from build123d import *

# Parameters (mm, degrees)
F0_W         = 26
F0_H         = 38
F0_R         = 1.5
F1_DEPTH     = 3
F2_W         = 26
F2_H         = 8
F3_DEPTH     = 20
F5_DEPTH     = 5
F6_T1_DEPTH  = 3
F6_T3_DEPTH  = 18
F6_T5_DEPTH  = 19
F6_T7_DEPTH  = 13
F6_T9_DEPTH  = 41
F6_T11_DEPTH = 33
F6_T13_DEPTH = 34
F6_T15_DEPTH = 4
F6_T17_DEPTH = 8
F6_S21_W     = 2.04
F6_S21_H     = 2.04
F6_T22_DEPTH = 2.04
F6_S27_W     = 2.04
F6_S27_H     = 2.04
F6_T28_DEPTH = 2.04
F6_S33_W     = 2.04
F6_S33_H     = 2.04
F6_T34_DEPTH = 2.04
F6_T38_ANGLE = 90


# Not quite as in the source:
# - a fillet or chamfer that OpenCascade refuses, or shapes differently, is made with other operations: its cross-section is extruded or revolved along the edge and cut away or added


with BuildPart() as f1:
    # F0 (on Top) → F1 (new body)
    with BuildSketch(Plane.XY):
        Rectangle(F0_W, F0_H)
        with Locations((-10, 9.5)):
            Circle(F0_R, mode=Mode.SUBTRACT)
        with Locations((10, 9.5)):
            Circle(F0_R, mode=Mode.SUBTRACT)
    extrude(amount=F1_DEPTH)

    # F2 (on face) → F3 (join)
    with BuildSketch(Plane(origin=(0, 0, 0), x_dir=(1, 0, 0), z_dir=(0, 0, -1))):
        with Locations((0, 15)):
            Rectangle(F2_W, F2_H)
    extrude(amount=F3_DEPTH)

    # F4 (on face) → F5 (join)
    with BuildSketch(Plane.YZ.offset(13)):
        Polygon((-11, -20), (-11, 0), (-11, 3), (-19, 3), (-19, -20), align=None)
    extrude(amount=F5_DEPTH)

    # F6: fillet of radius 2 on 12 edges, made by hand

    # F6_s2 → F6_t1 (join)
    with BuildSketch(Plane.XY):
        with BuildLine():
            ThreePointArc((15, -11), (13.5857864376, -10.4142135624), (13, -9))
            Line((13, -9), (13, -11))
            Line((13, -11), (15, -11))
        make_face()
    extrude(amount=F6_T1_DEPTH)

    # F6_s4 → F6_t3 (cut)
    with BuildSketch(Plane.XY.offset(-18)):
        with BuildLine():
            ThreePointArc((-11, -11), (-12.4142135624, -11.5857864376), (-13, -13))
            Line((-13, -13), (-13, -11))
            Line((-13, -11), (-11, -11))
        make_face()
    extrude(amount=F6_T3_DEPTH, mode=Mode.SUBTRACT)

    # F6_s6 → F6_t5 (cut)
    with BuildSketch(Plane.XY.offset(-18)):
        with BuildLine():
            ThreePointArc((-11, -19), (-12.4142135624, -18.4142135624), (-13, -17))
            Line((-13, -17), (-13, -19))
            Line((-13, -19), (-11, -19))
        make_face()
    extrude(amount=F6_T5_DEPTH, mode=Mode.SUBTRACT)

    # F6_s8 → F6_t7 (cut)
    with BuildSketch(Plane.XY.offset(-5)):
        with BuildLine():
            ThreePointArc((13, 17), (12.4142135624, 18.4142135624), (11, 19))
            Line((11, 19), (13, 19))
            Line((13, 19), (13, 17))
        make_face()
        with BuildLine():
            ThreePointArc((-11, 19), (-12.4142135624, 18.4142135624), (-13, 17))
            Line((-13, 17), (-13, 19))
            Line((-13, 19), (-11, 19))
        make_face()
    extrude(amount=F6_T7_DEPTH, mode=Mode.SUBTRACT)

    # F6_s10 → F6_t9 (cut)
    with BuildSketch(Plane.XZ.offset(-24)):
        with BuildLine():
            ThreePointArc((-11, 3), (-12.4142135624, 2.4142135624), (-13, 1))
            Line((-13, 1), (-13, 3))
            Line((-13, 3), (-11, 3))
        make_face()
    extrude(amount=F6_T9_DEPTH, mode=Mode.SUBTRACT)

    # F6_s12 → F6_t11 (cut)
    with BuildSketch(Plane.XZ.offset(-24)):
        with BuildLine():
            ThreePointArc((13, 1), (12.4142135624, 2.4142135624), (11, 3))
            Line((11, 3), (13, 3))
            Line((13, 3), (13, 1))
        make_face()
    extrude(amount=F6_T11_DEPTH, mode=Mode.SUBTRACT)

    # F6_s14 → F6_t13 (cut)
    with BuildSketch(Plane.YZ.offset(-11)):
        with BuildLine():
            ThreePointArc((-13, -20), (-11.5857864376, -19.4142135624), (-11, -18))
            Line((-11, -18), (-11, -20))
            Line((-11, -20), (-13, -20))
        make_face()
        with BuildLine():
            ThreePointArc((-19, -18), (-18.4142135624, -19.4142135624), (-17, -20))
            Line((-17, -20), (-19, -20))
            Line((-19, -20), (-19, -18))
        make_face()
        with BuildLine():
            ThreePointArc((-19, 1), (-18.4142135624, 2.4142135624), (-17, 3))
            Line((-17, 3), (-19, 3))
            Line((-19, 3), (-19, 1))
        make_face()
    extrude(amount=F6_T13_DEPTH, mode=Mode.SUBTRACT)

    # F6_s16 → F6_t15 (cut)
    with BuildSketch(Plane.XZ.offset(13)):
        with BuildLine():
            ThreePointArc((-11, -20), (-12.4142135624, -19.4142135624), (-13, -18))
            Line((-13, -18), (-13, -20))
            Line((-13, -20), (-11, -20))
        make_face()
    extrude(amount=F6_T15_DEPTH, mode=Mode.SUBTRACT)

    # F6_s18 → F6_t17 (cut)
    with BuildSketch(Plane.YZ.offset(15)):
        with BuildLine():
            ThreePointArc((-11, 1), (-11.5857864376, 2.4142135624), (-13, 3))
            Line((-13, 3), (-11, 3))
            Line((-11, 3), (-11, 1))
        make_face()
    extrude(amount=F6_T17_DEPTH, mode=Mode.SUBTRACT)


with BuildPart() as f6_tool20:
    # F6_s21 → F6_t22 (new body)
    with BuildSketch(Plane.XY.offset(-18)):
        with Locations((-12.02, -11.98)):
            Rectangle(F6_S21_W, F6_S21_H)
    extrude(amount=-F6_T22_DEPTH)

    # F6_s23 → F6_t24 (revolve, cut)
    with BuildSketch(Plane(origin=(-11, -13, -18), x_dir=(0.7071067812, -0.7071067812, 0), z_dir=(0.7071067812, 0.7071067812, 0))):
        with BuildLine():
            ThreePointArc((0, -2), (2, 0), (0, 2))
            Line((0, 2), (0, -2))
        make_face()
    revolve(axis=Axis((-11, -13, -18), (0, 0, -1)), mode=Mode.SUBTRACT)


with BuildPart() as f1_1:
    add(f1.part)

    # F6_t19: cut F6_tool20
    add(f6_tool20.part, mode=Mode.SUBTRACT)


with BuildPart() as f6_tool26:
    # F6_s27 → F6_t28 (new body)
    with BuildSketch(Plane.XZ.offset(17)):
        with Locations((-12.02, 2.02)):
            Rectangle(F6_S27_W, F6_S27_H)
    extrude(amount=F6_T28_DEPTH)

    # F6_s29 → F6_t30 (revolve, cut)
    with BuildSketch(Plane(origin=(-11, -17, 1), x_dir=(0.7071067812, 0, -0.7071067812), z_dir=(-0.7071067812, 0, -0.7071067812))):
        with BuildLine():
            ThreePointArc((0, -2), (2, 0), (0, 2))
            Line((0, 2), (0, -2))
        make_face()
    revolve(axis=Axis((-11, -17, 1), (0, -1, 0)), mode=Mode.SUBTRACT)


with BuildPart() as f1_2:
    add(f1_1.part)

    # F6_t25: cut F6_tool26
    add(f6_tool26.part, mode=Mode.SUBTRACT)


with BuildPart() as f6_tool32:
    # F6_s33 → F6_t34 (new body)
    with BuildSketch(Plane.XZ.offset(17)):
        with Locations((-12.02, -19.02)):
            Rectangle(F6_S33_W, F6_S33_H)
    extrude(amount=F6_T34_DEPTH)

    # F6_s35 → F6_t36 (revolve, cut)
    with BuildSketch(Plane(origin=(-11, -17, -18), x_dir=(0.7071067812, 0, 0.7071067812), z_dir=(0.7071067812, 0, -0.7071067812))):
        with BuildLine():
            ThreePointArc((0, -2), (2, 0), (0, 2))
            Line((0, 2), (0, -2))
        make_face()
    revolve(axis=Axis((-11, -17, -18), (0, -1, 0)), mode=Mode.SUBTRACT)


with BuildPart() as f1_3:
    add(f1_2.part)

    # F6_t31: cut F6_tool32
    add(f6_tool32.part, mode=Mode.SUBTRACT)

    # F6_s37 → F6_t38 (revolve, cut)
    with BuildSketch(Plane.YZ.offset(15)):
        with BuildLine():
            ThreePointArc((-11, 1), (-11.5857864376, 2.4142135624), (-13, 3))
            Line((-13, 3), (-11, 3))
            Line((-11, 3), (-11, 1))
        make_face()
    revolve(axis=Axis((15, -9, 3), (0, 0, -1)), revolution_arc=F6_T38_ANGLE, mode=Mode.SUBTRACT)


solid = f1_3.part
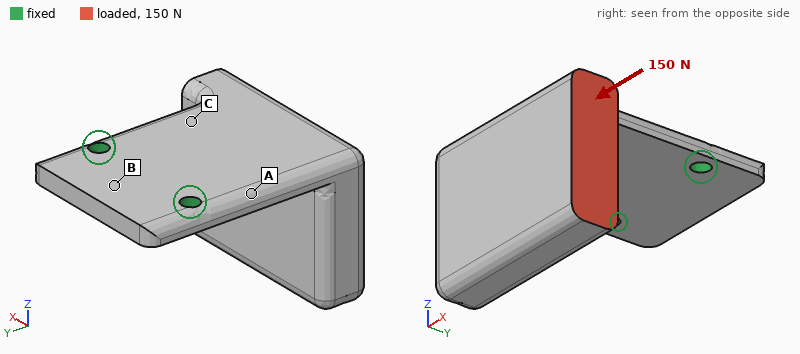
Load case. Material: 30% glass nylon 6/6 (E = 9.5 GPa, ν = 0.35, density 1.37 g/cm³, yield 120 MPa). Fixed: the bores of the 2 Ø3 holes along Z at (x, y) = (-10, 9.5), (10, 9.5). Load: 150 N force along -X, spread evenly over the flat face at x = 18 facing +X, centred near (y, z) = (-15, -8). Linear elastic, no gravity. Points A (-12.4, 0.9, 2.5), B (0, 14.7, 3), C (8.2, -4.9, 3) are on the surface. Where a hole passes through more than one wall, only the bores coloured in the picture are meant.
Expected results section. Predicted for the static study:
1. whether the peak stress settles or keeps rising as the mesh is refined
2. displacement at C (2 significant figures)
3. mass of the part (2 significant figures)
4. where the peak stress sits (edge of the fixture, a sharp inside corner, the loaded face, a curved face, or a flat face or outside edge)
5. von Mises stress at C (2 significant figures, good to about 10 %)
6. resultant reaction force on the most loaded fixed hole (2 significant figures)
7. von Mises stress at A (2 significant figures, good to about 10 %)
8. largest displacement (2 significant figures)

keeps rising
0.12 mm
11 g
edge of the fixture
20 MPa
210 N
22 MPa
0.61 mm
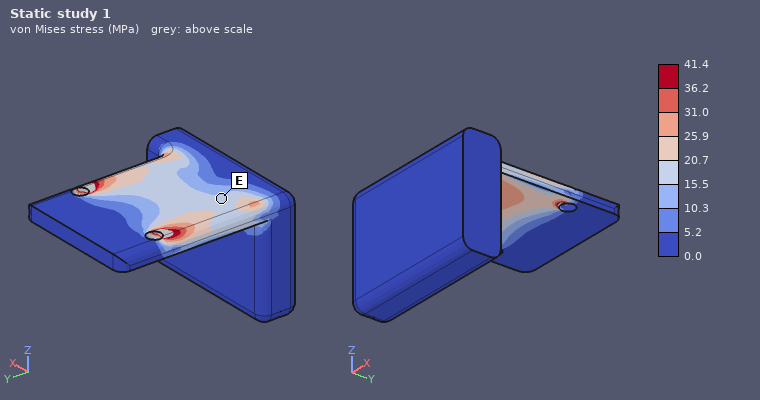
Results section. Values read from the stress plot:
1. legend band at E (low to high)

15.5 to 20.7 MPa
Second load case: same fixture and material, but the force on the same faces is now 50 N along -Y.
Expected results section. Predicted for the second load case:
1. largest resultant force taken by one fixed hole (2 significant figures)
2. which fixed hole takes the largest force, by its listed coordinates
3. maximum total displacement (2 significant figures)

69 N
(10, 9.5)
0.56 mm
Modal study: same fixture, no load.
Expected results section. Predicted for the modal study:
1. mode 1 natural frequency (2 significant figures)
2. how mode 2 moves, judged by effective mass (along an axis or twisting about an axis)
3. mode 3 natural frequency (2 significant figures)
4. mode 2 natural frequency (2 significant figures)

470 Hz
along X
2100 Hz
1000 Hz
